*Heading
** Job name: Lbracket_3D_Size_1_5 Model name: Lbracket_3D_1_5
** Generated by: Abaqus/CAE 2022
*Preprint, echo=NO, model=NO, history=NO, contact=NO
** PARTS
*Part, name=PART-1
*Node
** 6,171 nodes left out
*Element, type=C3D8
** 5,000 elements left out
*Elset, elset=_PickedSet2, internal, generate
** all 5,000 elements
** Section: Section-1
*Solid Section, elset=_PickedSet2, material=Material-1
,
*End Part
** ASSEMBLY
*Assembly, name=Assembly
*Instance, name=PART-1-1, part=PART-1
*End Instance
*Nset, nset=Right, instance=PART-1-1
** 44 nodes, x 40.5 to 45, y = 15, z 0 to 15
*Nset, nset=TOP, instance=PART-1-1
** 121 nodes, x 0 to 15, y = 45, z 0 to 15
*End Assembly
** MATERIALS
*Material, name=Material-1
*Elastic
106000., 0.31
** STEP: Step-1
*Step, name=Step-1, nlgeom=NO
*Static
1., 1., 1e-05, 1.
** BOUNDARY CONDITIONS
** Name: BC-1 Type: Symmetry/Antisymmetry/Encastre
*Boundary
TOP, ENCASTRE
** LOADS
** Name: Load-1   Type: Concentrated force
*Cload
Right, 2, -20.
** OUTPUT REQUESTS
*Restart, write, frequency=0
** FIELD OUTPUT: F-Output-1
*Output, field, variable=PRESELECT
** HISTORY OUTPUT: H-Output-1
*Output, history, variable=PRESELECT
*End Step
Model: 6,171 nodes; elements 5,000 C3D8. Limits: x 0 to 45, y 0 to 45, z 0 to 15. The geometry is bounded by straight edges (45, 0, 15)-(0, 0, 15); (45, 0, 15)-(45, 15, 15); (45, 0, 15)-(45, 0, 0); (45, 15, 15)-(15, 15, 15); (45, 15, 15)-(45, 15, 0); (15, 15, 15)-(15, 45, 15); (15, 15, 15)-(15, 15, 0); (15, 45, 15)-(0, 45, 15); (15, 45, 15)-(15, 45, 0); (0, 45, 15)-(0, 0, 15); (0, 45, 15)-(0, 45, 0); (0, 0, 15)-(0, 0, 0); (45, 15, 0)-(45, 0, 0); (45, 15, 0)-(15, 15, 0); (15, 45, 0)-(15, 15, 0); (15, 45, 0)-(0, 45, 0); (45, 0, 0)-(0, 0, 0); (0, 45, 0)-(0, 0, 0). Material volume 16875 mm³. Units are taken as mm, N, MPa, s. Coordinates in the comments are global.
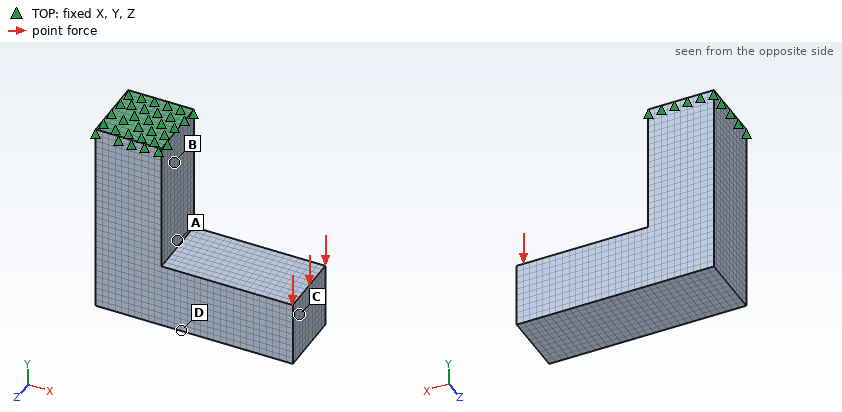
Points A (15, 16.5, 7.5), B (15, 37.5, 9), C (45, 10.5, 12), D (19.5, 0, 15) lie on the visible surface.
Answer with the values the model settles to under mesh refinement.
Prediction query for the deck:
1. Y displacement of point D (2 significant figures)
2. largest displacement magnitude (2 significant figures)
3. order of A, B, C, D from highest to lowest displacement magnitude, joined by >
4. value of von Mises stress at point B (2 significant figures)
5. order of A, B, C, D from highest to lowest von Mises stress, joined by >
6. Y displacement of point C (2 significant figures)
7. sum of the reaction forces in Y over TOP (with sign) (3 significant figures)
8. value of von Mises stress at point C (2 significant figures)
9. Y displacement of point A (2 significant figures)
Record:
-0.032 mm
0.14 mm
C > D > A > B
59 MPa
A > B > D > C
-0.12 mm
880 N
13 MPa
-0.016 mm
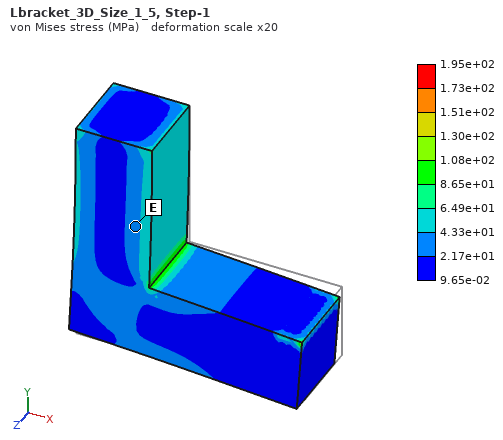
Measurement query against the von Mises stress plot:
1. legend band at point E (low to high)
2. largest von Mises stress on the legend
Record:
2.17e+01 to 4.33e+01 MPa
1.95e+02 MPa
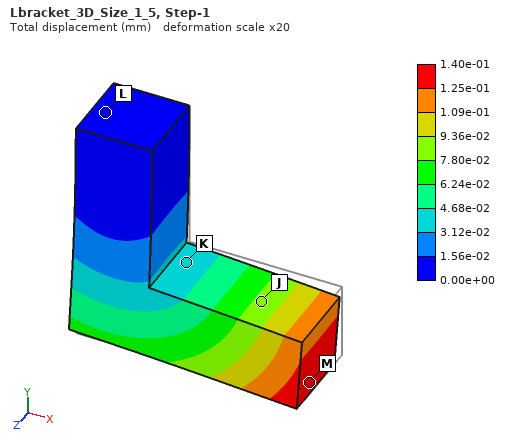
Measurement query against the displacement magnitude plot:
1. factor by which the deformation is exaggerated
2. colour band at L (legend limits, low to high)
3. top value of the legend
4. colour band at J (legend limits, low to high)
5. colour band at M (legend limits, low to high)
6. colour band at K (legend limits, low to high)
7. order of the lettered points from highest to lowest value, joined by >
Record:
20
0.00e+00 to 1.56e-02 mm
1.40e-01 mm
7.80e-02 to 9.36e-02 mm
1.25e-01 to 1.40e-01 mm
3.12e-02 to 4.68e-02 mm
M > J > K > L
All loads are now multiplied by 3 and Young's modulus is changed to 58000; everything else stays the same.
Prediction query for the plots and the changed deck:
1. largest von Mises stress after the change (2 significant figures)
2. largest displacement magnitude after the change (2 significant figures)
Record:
580 MPa
0.77 mm
